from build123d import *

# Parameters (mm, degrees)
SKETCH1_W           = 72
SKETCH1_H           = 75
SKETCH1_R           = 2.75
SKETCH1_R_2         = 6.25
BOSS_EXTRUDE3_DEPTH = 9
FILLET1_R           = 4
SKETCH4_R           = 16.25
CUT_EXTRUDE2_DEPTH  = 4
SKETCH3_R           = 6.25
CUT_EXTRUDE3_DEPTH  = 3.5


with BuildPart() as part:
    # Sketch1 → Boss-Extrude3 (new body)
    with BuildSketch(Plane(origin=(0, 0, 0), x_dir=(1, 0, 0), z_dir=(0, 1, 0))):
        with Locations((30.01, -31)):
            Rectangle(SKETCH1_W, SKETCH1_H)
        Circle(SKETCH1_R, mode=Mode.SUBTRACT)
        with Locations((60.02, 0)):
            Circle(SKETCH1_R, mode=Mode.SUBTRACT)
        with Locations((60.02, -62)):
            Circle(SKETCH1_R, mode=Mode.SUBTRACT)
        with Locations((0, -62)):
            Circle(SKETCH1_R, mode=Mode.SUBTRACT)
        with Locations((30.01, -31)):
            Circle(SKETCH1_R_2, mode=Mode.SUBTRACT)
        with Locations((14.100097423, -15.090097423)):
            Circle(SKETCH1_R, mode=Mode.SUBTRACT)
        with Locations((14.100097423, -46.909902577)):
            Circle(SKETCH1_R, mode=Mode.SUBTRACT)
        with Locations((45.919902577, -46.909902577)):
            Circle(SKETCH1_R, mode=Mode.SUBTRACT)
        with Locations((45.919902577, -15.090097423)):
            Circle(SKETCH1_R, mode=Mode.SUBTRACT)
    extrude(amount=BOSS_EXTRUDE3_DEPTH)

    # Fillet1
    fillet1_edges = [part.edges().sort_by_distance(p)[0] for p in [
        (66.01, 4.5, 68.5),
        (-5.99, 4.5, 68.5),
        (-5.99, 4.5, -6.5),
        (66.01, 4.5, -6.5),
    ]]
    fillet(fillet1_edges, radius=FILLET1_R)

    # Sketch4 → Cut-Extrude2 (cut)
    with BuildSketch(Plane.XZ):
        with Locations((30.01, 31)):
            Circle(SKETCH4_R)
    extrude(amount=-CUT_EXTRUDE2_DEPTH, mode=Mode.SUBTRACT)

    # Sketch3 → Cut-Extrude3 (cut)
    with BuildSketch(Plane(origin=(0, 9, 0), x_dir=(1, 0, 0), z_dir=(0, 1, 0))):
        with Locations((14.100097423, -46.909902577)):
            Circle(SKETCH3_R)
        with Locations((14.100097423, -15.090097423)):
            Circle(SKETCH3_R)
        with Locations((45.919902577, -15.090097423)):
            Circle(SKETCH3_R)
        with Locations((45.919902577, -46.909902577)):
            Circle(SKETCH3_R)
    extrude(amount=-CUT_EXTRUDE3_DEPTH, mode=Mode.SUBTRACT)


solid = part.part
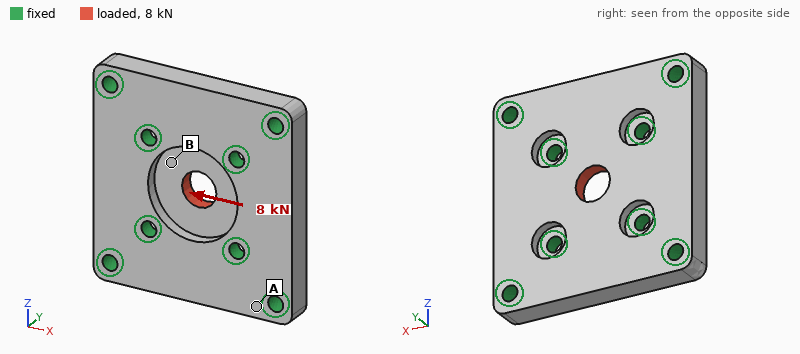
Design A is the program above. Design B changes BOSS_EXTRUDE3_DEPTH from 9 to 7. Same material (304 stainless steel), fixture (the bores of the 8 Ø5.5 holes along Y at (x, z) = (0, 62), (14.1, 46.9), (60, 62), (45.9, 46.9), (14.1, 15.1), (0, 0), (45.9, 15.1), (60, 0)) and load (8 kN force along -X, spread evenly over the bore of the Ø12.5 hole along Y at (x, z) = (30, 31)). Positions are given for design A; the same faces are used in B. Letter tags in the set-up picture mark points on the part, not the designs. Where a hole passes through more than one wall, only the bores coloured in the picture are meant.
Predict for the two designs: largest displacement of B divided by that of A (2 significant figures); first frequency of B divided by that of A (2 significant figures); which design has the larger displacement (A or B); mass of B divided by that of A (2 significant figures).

1.5
0.89
B
0.77
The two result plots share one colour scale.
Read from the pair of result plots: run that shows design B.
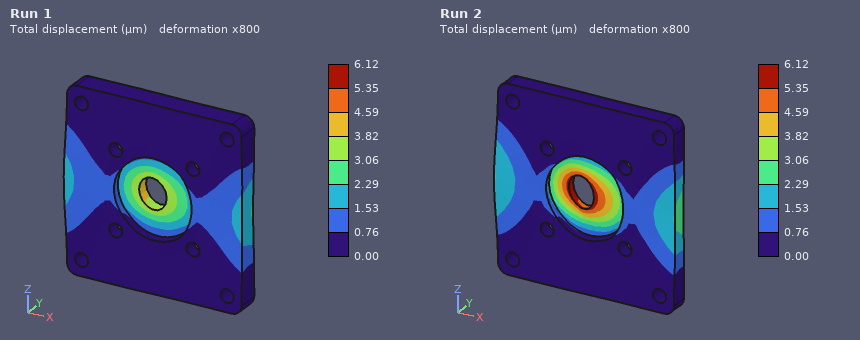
Run 2
